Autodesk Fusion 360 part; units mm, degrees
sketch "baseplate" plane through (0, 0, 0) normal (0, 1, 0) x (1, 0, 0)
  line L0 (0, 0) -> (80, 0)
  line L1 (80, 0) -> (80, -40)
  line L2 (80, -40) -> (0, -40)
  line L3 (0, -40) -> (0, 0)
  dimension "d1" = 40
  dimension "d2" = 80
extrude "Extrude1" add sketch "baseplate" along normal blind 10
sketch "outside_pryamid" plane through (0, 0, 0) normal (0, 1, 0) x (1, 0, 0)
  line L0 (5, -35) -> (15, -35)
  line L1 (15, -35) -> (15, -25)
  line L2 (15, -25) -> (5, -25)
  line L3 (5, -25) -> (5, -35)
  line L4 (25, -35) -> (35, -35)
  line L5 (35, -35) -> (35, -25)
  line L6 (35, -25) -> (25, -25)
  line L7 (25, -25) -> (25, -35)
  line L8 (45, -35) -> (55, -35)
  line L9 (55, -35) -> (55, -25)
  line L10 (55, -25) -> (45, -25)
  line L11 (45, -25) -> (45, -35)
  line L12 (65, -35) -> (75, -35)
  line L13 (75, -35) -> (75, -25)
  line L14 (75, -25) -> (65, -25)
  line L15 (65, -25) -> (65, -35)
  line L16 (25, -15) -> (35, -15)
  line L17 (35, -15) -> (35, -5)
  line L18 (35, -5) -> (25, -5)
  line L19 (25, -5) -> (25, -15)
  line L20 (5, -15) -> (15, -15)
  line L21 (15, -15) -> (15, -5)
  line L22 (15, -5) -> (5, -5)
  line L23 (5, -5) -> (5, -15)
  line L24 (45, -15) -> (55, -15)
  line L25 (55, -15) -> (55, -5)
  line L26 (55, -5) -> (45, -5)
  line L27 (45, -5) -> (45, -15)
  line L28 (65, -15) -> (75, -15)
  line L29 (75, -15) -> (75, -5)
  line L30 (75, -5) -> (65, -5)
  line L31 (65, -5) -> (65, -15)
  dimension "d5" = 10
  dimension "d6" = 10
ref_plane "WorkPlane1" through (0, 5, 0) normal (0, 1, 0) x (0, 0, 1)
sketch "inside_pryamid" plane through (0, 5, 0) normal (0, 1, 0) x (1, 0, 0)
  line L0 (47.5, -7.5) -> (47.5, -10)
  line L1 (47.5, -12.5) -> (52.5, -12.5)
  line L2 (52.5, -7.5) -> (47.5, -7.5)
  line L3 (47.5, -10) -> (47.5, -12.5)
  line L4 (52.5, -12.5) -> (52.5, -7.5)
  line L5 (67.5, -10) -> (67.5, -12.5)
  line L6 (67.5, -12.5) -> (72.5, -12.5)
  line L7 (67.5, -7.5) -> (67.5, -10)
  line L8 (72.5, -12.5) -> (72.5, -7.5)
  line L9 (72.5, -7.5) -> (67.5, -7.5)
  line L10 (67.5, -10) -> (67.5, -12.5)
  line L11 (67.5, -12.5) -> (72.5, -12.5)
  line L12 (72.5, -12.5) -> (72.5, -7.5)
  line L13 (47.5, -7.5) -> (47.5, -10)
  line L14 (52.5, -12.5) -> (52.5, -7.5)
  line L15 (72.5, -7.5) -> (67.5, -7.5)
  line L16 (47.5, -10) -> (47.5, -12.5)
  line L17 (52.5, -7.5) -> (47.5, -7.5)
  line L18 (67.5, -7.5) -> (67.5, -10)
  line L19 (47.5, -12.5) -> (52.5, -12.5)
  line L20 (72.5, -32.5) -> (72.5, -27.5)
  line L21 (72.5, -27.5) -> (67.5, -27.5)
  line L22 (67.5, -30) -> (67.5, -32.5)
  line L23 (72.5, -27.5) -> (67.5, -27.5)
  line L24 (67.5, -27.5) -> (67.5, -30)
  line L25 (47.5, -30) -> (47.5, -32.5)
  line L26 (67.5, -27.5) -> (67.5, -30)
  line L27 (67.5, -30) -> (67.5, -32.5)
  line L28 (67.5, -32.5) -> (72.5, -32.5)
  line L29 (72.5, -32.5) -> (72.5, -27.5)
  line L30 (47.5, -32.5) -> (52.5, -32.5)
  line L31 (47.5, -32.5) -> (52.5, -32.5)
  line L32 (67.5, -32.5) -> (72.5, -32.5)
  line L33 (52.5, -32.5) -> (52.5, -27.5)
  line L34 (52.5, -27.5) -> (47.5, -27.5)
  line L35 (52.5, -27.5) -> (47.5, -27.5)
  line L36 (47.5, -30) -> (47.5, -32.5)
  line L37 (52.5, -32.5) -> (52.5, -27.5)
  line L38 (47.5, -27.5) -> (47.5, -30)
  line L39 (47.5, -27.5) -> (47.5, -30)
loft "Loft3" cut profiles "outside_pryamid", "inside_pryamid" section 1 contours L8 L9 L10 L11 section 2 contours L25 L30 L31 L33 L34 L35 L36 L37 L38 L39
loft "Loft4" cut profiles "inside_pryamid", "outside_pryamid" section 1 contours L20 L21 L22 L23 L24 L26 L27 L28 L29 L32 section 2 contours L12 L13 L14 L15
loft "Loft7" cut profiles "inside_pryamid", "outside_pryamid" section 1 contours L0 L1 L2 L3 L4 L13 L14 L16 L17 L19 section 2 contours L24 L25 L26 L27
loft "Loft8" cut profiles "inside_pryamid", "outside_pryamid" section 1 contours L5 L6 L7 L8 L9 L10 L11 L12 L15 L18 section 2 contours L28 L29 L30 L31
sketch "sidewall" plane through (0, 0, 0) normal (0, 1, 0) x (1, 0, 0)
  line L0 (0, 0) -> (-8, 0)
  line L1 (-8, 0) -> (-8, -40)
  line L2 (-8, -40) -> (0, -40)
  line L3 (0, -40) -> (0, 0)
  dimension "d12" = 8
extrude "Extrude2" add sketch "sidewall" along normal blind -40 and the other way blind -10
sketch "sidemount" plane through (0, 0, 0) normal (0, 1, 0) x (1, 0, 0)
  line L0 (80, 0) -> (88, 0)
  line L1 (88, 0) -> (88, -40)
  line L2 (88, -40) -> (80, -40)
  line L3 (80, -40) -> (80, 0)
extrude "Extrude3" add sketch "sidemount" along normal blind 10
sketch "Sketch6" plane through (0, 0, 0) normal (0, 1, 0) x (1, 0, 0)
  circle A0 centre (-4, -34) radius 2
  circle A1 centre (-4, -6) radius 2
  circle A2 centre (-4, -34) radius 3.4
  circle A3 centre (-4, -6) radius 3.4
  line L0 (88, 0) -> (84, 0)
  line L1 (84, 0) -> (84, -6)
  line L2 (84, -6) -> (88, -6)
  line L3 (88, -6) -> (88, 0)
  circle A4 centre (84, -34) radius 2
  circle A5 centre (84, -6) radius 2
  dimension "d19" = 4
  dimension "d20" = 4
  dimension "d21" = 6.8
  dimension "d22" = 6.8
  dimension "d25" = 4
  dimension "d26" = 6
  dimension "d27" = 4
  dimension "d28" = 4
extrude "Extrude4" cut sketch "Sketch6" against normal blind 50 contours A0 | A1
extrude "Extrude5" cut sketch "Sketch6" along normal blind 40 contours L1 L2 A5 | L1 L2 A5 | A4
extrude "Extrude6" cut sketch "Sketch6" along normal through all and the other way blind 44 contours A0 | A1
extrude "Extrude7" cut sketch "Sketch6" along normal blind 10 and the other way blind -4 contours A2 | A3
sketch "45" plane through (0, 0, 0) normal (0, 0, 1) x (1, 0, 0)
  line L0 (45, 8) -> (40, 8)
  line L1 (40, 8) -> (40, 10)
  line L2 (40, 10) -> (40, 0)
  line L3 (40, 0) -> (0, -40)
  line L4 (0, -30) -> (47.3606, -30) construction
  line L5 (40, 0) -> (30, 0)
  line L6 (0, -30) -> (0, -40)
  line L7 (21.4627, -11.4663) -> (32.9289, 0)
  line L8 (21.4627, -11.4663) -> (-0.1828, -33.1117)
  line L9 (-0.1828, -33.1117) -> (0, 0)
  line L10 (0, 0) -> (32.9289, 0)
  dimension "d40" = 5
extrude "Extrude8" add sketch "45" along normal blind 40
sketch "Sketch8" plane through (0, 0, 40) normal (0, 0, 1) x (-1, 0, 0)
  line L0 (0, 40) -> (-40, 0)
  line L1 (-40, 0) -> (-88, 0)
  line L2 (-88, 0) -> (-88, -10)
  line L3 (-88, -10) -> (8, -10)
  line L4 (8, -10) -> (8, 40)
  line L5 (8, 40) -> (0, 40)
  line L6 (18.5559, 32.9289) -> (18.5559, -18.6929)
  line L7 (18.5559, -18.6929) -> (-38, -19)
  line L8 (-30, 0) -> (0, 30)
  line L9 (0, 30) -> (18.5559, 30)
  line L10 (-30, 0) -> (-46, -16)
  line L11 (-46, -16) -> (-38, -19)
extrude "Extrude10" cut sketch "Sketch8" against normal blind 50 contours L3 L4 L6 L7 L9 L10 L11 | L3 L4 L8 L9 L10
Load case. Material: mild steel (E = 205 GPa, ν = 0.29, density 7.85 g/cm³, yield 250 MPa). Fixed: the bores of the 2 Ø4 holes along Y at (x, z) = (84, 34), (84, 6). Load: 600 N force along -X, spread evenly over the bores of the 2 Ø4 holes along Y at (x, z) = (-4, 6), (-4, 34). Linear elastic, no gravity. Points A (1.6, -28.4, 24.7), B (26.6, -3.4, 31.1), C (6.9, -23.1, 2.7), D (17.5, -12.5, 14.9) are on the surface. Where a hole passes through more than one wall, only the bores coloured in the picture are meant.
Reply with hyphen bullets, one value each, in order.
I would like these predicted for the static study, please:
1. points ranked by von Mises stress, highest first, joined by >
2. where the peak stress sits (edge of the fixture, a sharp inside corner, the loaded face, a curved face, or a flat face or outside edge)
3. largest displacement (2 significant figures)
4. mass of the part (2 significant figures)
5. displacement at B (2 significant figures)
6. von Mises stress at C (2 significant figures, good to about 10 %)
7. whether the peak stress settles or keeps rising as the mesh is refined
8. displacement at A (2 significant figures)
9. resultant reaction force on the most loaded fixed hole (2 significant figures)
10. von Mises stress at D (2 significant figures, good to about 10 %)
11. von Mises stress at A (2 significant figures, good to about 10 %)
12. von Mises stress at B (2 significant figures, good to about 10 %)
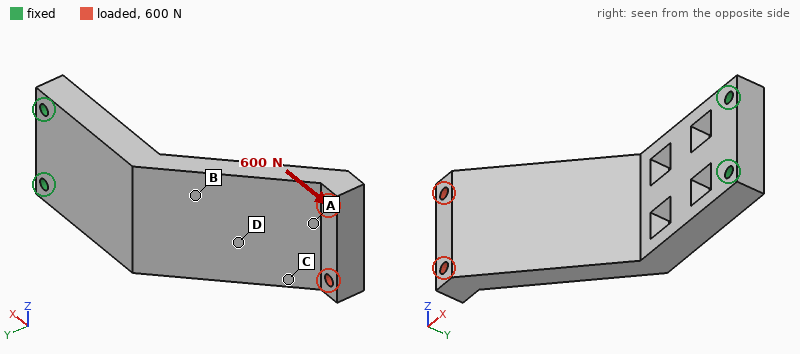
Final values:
- B > D > C > A
- edge of the fixture
- 0.29 mm
- 290 g
- 0.086 mm
- 15 MPa
- keeps rising
- 0.22 mm
- 300 N
- 33 MPa
- 7.0 MPa
- 49 MPa
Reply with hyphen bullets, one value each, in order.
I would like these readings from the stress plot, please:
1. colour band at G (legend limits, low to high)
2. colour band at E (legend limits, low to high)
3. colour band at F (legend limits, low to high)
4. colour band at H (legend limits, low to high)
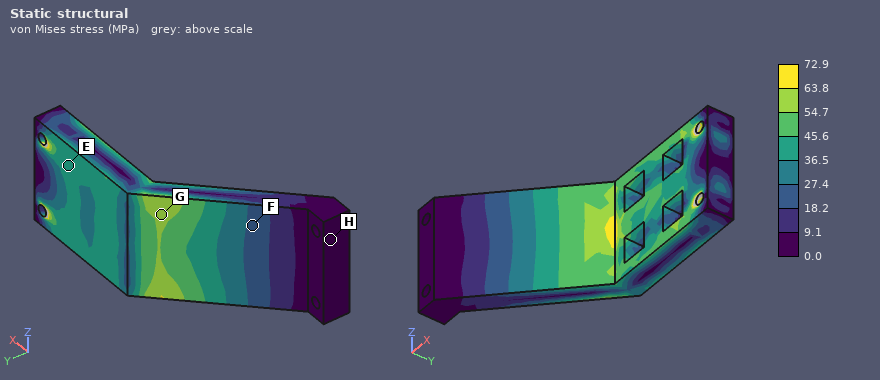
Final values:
- 54.7 to 63.8 MPa
- 36.5 to 45.6 MPa
- 18.2 to 27.4 MPa
- 0.0 to 9.1 MPa
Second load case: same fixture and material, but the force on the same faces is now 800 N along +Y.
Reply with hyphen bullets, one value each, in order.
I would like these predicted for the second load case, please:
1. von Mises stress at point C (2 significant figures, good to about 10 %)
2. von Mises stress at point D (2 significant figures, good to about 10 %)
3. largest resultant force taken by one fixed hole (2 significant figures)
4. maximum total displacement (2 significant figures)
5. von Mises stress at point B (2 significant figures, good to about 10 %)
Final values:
- 35 MPa
- 57 MPa
- 410 N
- 0.58 mm
- 79 MPa
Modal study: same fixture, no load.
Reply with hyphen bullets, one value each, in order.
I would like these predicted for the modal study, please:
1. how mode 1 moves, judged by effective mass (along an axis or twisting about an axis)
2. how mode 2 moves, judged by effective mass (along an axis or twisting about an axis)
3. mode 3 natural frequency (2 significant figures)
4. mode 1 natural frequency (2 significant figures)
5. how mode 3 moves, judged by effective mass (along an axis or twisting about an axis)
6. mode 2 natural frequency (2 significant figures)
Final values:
- along Y
- along Z
- 2800 Hz
- 690 Hz
- along Y
- 1700 Hz
